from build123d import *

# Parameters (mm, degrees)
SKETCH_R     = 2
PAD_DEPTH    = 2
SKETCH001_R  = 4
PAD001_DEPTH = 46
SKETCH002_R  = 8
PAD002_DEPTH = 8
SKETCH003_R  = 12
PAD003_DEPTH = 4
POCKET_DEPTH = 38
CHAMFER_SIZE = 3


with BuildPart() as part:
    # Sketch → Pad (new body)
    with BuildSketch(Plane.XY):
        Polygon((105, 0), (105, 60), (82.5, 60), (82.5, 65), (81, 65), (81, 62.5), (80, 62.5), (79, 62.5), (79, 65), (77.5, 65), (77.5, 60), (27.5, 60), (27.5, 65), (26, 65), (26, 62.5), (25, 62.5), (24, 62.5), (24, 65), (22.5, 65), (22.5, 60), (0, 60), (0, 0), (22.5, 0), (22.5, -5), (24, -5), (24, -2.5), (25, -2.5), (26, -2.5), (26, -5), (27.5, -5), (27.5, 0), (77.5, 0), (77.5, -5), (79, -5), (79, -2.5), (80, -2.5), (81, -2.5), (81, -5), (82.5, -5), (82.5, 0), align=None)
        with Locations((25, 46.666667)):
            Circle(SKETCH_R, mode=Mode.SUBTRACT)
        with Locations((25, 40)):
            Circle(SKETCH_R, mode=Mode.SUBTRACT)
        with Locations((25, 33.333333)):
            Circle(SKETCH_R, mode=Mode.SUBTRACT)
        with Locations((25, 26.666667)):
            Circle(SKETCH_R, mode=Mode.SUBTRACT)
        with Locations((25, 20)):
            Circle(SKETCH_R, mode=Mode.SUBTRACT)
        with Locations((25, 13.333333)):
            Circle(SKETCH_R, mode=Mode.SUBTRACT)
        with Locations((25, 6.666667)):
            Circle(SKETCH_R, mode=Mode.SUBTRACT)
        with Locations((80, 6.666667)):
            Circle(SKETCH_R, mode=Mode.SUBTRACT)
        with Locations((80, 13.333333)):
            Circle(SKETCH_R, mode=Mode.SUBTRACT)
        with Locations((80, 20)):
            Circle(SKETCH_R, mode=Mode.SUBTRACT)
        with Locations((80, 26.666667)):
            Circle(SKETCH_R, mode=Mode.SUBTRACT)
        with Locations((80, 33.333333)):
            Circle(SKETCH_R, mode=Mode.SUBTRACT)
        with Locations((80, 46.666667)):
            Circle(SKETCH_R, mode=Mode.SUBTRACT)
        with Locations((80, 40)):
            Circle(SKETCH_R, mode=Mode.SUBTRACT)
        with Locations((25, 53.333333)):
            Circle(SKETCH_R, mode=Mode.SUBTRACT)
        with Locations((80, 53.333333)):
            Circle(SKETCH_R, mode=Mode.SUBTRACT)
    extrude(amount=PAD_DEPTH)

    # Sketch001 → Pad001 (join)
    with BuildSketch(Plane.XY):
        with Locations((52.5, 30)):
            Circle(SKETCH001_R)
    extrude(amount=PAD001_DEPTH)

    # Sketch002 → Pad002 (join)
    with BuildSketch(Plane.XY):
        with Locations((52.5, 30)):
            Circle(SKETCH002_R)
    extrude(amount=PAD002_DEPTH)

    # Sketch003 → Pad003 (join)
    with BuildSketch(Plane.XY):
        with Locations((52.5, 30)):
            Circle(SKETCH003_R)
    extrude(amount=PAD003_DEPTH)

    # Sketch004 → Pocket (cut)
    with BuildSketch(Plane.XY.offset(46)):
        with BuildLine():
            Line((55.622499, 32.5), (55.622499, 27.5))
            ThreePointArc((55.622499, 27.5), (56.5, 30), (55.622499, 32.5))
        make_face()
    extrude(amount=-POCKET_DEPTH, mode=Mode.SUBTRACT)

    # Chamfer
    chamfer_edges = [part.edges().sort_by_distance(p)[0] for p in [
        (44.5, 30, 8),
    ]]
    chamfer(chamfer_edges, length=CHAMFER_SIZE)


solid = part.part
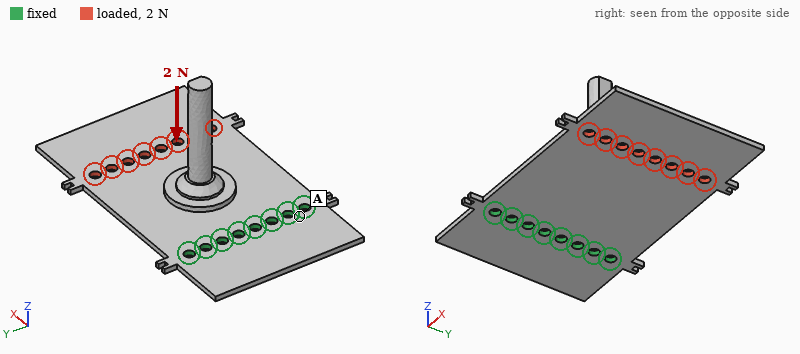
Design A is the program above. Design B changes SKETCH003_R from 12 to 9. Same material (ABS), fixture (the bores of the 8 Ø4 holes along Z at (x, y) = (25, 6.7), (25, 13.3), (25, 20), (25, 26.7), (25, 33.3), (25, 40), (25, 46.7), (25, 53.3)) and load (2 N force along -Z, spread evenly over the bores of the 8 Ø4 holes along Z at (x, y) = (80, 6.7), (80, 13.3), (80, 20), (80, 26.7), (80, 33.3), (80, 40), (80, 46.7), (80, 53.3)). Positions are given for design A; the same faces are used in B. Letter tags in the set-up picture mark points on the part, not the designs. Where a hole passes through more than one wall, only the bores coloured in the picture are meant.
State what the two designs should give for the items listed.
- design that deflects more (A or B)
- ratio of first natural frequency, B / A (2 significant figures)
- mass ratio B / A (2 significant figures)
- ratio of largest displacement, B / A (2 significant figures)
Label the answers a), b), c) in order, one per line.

a) B
b) 0.96
c) 0.97
d) 1.1
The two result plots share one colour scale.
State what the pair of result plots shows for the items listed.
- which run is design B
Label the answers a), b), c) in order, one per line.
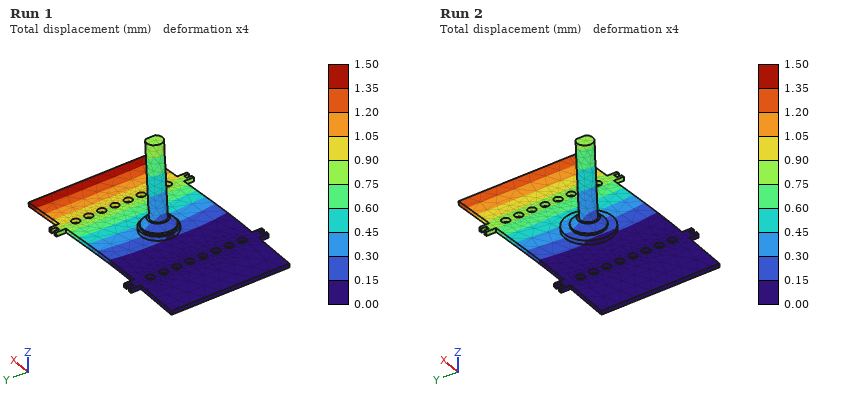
a) Run 1
